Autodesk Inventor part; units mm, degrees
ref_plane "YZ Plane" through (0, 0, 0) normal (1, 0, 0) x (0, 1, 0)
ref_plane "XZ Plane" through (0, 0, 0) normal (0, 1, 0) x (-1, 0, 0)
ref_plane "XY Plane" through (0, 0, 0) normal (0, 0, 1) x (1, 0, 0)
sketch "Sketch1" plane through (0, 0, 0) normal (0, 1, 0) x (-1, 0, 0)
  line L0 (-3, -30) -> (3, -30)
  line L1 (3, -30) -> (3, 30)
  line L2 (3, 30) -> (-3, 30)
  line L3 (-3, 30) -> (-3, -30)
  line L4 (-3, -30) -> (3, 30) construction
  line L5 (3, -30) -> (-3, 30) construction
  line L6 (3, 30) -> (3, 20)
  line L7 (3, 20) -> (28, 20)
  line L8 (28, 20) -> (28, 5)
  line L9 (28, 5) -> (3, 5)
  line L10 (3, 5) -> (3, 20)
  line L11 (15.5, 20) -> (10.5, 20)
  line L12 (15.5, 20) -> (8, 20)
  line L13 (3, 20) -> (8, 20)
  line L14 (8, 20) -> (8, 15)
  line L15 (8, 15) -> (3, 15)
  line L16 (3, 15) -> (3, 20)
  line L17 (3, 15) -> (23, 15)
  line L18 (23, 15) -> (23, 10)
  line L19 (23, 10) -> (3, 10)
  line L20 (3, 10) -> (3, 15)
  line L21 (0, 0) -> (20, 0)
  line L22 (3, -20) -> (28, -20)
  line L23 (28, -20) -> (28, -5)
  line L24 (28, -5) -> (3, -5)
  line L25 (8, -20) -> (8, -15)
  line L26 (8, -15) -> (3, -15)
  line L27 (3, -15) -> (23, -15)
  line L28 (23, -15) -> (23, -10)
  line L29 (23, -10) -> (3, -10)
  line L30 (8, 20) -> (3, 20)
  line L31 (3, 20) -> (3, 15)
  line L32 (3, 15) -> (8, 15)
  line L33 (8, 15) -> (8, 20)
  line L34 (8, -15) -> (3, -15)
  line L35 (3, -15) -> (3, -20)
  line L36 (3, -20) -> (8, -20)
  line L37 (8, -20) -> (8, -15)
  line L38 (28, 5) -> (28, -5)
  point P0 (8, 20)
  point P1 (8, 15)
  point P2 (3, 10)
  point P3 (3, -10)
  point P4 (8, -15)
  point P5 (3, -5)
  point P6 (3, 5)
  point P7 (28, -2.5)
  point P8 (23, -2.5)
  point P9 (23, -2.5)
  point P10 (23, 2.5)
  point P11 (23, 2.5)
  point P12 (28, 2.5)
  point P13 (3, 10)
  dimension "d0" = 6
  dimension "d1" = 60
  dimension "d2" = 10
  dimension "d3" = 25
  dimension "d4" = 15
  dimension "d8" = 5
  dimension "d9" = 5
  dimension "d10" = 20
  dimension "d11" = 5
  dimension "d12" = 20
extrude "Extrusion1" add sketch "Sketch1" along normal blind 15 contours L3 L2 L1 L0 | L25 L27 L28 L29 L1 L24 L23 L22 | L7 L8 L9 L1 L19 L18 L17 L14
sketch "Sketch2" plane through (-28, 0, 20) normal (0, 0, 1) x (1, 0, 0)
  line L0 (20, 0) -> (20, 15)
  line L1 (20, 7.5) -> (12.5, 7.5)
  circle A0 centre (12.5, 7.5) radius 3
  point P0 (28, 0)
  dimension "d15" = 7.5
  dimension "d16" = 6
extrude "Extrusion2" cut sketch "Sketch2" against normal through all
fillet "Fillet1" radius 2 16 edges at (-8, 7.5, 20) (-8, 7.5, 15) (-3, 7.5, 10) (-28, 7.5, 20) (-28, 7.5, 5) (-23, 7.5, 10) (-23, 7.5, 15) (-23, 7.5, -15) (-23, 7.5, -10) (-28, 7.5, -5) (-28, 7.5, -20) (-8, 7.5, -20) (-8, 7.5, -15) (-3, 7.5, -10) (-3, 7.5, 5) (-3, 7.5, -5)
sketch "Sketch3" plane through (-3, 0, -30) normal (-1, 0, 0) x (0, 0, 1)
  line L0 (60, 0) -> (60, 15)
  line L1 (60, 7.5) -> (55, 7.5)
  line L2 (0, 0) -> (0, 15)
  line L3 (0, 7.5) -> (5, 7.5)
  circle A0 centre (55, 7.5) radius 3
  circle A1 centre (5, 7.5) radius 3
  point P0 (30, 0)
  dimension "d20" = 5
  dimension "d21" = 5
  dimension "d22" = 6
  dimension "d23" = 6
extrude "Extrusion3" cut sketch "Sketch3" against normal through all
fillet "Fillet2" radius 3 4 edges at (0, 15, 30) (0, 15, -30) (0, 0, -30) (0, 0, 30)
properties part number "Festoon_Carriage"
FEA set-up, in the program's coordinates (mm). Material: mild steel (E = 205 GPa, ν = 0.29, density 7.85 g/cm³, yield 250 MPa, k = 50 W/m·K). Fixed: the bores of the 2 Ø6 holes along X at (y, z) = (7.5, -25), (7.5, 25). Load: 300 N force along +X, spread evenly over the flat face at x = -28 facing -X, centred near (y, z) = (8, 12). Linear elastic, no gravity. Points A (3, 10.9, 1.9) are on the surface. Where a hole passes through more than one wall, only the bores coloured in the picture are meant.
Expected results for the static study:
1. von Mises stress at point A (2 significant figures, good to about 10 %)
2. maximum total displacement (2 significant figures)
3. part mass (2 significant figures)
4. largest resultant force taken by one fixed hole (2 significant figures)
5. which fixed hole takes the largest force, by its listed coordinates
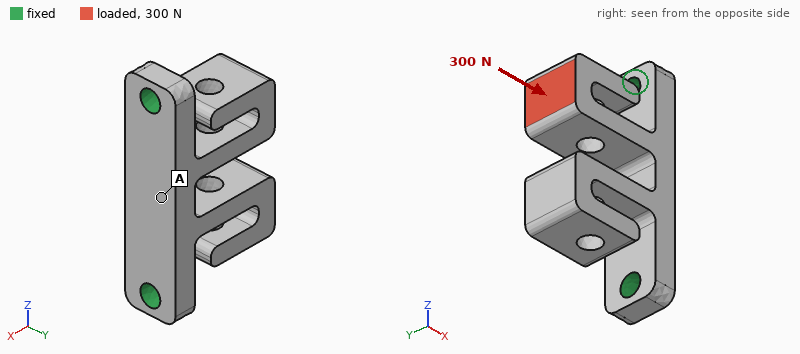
4.6 MPa
24 µm
94 g
260 N
(7.5, 25)
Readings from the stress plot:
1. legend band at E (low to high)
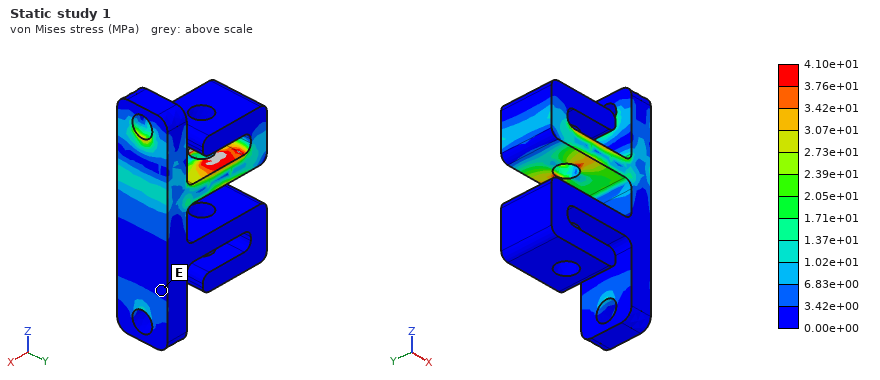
0.00e+00 to 3.42e+00 MPa
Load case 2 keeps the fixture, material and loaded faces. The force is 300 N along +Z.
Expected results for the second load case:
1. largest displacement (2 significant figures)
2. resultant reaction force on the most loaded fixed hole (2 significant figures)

82 µm
290 N
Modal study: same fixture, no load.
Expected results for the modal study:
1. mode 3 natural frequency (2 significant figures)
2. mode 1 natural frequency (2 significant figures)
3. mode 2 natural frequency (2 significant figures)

3000 Hz
2900 Hz
3000 Hz
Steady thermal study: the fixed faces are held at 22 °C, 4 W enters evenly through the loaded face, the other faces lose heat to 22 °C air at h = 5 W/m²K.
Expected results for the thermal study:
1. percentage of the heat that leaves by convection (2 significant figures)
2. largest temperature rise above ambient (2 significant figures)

9.0 %
39 K
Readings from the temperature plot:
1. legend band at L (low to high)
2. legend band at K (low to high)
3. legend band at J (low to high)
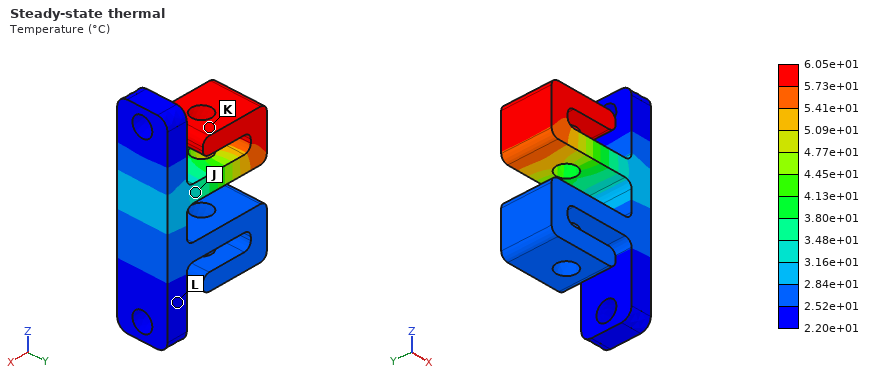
2.20e+01 to 2.52e+01 °C
5.73e+01 to 6.05e+01 °C
3.16e+01 to 3.48e+01 °C
